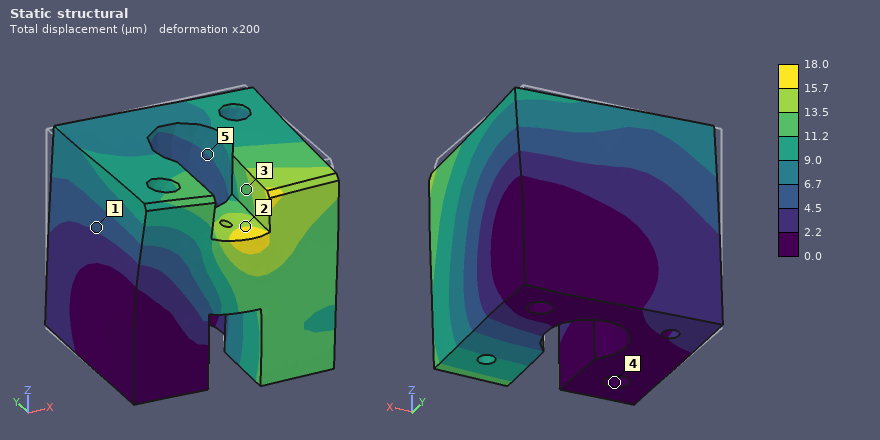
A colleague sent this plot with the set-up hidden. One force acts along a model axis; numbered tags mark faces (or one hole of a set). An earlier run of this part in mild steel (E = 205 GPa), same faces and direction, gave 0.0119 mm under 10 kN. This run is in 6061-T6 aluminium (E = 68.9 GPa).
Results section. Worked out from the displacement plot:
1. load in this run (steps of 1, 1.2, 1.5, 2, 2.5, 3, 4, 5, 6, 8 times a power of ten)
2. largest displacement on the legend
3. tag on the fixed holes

5 kN
18.0 µm
4
